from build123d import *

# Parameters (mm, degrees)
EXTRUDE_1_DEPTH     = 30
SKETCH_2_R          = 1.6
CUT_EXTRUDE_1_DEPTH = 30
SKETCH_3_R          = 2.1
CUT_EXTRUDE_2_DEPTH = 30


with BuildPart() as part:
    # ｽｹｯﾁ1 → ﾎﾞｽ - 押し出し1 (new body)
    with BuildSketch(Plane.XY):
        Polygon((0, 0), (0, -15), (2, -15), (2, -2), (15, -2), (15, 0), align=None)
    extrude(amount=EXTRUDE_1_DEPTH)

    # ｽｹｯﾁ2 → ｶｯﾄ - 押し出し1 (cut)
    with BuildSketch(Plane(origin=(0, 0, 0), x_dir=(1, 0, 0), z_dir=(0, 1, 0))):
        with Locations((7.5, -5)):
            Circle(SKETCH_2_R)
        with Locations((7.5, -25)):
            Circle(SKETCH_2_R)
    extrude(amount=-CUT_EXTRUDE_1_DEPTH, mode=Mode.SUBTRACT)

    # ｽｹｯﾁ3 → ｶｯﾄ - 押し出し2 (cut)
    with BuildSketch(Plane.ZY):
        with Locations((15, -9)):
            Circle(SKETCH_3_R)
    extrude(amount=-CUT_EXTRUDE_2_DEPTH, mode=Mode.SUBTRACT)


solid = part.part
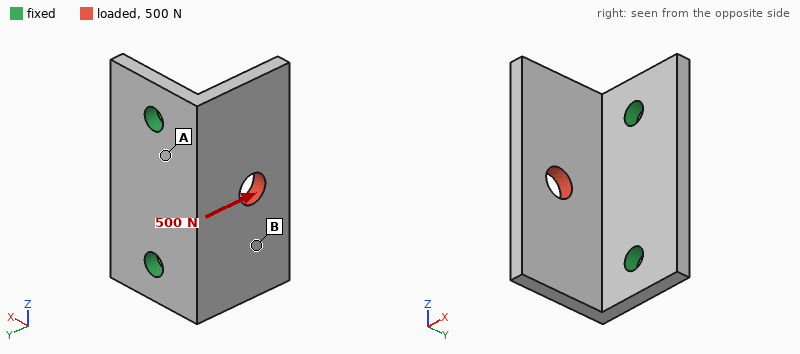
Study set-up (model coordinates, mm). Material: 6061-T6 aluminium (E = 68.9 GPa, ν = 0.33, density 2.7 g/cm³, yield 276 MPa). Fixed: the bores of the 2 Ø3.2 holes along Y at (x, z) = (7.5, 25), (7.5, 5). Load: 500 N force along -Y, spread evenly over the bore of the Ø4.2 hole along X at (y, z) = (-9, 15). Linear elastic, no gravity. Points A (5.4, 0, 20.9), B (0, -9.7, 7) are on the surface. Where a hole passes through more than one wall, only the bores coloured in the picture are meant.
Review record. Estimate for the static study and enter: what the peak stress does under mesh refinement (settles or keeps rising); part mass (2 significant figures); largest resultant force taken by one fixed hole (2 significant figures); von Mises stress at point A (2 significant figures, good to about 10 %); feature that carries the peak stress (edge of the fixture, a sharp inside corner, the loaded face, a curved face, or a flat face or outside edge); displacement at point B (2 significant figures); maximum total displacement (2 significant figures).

keeps rising
4.4 g
260 N
67 MPa
edge of the fixture
0.072 mm
0.11 mm
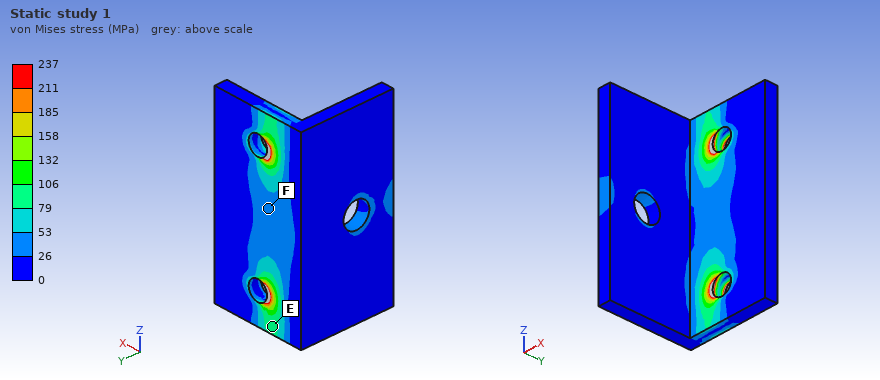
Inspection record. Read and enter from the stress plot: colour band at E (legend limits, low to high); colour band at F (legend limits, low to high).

79 to 106 MPa
26 to 53 MPa
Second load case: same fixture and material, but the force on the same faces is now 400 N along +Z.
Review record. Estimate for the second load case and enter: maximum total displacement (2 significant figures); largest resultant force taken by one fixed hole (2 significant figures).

40 µm
270 N
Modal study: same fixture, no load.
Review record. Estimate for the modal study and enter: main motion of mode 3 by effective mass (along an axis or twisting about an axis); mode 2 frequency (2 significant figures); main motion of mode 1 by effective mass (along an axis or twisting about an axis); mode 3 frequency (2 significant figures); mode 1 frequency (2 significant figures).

along Z
8800 Hz
along X
16 kHz
5100 Hz
